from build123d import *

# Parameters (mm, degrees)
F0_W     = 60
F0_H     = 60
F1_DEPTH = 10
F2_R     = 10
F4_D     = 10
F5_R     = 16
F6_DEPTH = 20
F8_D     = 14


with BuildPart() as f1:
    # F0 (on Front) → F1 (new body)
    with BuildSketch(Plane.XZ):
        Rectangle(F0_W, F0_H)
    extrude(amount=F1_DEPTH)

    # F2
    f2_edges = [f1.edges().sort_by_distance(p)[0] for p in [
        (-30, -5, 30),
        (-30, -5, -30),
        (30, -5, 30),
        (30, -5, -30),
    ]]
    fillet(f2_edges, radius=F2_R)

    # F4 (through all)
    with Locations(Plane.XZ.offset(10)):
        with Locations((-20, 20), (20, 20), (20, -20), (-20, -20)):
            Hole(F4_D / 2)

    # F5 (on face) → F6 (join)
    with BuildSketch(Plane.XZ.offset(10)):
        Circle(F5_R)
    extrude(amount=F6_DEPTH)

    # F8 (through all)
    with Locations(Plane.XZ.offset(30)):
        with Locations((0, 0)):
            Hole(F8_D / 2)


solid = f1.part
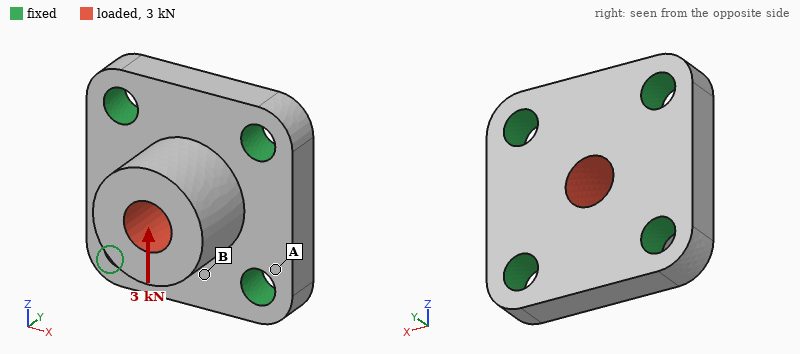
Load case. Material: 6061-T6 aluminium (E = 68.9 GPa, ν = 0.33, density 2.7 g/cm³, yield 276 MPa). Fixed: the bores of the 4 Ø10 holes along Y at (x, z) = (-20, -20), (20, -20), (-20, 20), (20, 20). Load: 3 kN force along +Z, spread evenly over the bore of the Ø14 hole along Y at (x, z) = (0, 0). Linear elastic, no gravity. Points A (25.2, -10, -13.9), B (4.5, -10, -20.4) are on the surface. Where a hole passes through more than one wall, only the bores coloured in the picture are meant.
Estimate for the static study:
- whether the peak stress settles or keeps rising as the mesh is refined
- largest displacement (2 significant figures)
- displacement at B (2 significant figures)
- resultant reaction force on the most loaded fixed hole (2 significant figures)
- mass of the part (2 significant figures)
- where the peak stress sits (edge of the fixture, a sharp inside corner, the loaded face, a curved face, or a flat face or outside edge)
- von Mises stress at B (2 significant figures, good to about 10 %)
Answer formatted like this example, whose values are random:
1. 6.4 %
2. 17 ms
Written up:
1. keeps rising
2. 6.6 µm
3. 1.5 µm
4. 930 N
5. 120 g
6. edge of the fixture
7. 3.7 MPa
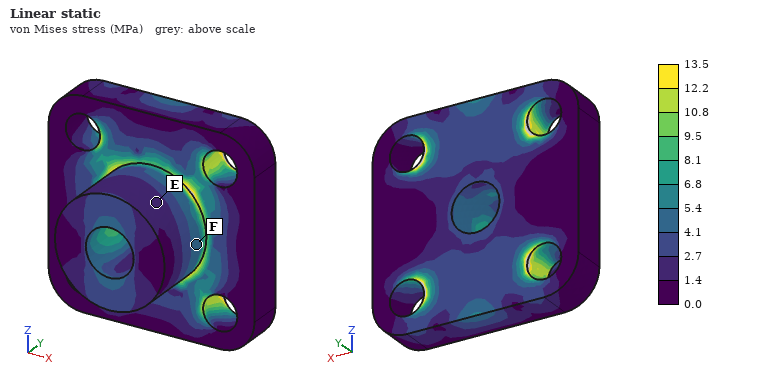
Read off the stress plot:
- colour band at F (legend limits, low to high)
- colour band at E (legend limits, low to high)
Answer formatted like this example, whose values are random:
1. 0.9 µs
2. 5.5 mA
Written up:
1. 4.1 to 5.4 MPa
2. 1.4 to 2.7 MPa
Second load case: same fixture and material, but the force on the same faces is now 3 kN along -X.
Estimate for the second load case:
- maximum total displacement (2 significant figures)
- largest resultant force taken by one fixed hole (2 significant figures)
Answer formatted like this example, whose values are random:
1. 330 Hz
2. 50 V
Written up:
1. 6.6 µm
2. 930 N
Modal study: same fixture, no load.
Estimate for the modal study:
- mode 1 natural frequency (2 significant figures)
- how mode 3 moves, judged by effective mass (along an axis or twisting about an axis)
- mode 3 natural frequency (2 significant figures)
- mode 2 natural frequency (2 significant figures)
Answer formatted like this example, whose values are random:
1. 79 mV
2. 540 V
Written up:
1. 17 kHz
2. along Y
3. 19 kHz
4. 17 kHz
